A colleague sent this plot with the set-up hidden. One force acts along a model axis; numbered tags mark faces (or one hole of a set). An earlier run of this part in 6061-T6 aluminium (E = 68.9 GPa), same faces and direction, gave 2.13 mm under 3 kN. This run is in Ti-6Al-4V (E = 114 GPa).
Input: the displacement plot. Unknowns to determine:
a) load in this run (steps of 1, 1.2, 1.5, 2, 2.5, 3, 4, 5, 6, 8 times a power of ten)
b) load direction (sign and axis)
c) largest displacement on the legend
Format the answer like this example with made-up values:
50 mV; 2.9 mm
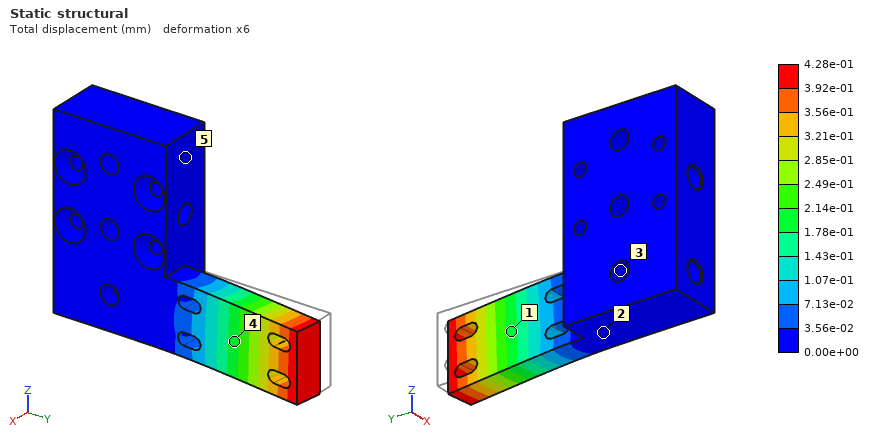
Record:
1 kN; +X; 4.28e-01 mm
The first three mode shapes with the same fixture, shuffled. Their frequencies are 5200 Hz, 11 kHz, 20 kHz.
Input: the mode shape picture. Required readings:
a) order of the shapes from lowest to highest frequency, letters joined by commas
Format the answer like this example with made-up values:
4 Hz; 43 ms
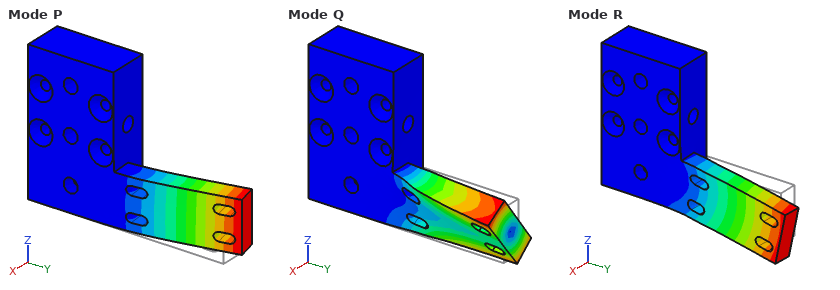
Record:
P, R, Q
